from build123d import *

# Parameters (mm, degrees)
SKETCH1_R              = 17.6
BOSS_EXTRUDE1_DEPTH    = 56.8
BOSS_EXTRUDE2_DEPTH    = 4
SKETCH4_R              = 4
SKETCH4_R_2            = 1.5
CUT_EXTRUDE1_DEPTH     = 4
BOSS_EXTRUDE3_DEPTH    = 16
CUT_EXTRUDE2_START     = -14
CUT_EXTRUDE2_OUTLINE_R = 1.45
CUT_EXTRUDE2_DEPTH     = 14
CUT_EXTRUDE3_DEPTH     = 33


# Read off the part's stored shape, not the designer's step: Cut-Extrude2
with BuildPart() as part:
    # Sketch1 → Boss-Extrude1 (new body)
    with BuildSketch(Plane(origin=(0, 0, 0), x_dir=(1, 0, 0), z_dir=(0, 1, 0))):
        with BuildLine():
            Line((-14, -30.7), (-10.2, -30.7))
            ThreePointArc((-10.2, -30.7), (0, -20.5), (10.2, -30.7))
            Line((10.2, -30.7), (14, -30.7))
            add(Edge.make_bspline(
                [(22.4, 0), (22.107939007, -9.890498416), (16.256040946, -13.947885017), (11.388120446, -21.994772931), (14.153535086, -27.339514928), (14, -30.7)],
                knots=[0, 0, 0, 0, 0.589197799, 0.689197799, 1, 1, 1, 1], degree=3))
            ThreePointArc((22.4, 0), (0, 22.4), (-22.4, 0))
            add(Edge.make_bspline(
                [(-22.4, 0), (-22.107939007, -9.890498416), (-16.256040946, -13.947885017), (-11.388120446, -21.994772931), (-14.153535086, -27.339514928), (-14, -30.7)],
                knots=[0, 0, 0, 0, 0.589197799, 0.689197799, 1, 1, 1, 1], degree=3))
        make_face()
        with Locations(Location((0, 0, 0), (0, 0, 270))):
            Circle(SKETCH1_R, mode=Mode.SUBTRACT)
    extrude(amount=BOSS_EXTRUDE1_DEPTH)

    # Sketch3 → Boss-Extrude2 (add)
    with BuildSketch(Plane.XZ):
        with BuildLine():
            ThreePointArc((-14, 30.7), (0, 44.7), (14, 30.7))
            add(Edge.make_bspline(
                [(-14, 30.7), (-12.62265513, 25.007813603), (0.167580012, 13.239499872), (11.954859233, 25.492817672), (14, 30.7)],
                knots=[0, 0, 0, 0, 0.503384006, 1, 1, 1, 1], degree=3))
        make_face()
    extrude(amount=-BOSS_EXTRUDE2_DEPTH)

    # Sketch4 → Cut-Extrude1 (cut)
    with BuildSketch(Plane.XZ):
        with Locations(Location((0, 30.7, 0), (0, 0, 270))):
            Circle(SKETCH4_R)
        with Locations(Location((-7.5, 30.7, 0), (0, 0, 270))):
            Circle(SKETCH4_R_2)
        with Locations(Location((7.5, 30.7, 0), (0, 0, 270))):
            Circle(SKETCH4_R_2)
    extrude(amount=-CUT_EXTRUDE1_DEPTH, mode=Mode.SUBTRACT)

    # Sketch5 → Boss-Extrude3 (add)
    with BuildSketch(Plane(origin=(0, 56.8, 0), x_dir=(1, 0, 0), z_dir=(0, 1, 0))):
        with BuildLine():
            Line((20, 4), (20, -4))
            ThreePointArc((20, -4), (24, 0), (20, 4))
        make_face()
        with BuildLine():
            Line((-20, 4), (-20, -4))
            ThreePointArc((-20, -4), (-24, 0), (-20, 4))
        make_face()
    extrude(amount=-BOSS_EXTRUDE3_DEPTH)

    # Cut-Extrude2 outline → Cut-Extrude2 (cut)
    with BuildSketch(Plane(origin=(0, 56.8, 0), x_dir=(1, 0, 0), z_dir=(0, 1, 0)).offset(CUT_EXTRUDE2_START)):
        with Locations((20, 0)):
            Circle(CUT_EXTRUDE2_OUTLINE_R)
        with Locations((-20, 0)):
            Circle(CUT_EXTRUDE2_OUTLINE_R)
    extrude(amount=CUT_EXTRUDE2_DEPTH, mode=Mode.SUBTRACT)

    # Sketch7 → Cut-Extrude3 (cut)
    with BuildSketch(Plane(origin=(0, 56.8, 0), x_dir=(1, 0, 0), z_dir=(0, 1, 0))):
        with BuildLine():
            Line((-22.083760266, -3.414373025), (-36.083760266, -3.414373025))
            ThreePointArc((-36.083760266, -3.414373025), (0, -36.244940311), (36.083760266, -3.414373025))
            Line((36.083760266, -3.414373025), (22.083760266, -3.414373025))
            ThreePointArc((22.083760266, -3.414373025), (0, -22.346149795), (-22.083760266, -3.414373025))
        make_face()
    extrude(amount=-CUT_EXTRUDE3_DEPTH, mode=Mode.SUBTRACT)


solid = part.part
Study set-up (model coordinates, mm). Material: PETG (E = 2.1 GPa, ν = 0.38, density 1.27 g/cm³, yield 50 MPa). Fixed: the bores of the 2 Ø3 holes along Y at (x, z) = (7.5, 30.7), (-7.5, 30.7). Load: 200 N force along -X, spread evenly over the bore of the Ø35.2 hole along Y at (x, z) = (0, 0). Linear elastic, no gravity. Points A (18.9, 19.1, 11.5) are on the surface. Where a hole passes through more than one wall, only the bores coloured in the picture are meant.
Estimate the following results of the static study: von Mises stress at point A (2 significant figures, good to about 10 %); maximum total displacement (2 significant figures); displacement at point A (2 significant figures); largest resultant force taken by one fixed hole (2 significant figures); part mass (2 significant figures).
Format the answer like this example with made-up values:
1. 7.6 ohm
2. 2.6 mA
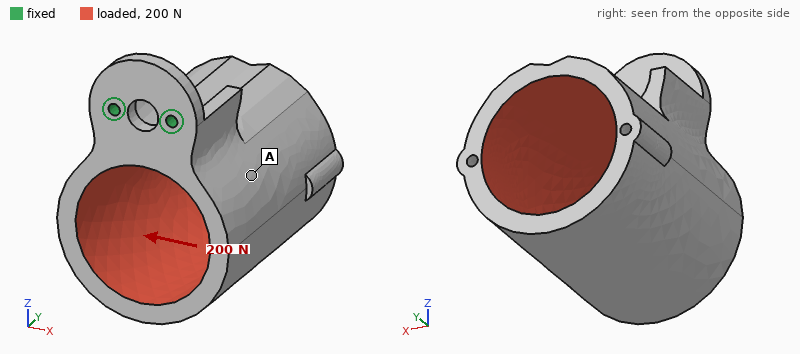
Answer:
1. 2.8 MPa
2. 1.2 mm
3. 0.43 mm
4. 450 N
5. 47 g
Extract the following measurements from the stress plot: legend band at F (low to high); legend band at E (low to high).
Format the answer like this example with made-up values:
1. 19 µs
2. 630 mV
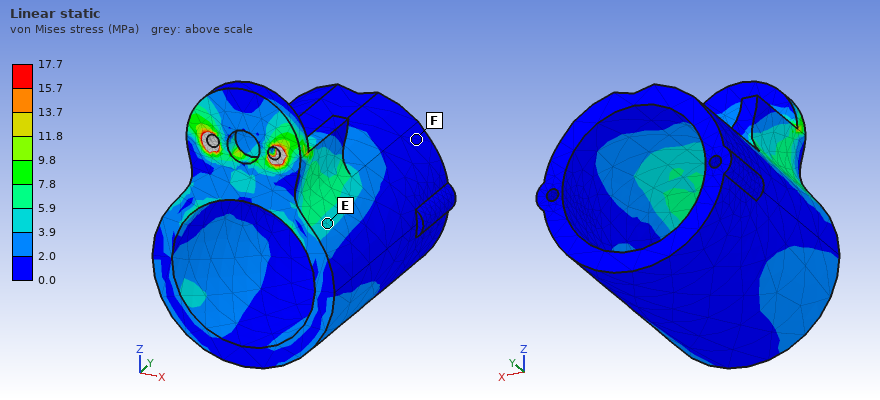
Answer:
1. 0.0 to 2.0 MPa
2. 3.9 to 5.9 MPa
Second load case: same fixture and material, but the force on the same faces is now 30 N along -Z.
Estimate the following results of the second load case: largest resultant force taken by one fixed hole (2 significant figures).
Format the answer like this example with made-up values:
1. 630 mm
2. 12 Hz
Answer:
1. 15 N
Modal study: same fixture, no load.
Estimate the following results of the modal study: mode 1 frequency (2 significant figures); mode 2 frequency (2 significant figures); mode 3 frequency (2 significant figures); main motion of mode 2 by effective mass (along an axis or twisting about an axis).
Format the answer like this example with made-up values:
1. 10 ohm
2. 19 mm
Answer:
1. 130 Hz
2. 380 Hz
3. 480 Hz
4. along X
